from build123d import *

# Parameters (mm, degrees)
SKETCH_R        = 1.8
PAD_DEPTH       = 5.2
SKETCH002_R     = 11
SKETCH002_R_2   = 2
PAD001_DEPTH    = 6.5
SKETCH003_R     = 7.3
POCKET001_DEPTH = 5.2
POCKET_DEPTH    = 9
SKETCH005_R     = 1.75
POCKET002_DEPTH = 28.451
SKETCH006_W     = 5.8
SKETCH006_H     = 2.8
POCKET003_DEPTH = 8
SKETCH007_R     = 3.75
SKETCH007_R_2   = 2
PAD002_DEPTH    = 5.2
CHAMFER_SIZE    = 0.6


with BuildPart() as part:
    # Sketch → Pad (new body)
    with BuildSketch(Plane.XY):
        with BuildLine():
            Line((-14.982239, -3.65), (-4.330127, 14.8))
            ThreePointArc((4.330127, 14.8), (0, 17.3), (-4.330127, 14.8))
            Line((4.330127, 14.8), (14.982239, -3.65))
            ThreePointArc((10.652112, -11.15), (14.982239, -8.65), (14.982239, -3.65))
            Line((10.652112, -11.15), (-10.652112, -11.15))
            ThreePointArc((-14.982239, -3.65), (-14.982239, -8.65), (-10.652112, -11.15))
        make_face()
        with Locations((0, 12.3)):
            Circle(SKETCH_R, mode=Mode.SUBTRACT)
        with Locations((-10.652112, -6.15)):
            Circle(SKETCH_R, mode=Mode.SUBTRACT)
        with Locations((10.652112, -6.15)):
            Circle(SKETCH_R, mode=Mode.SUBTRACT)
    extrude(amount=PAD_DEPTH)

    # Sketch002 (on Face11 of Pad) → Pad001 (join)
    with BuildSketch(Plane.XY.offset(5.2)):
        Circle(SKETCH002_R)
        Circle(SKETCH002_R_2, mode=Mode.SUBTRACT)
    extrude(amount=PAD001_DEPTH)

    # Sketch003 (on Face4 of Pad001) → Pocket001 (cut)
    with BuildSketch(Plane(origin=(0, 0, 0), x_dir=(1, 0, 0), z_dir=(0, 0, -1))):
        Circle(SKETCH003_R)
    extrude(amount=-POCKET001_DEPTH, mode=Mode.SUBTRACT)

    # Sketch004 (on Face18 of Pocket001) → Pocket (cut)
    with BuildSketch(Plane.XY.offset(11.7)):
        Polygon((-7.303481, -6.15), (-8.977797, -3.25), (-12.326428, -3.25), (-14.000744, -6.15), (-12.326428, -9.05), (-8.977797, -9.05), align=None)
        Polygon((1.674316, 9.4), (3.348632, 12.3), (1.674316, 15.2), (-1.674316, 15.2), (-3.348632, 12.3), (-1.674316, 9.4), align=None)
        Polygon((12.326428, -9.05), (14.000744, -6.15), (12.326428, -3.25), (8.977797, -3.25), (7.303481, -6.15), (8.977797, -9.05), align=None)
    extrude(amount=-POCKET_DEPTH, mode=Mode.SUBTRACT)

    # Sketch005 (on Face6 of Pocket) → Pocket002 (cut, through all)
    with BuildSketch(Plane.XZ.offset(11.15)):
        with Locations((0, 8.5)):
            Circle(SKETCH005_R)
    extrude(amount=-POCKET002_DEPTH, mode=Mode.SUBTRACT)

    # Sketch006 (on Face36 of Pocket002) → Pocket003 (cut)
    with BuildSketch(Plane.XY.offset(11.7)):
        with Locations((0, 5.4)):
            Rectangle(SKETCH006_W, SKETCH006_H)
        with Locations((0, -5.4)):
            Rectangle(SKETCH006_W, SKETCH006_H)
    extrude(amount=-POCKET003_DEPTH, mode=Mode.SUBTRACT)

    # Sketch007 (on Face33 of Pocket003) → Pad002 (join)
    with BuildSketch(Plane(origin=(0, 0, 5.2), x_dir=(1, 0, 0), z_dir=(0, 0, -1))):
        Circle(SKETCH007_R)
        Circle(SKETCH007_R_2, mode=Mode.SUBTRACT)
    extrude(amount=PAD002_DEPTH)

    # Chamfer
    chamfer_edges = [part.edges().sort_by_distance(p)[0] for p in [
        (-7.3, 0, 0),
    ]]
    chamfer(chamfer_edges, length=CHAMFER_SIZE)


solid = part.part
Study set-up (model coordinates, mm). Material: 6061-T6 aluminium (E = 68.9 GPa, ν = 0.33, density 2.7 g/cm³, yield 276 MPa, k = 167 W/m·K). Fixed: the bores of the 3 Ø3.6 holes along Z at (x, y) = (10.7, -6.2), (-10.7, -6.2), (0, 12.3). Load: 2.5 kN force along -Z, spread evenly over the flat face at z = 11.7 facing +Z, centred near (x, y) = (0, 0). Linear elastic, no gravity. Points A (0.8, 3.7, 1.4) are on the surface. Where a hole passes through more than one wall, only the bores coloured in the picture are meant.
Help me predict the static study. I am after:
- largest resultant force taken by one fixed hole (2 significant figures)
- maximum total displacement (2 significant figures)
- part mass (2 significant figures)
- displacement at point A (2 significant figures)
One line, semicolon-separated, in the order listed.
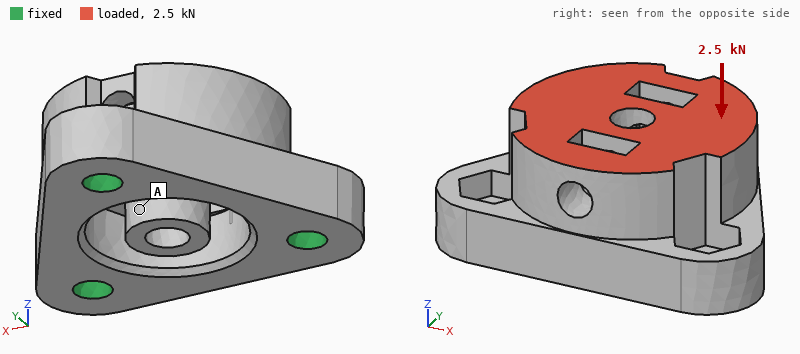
920 N; 8.2 µm; 11 g; 7.1 µm
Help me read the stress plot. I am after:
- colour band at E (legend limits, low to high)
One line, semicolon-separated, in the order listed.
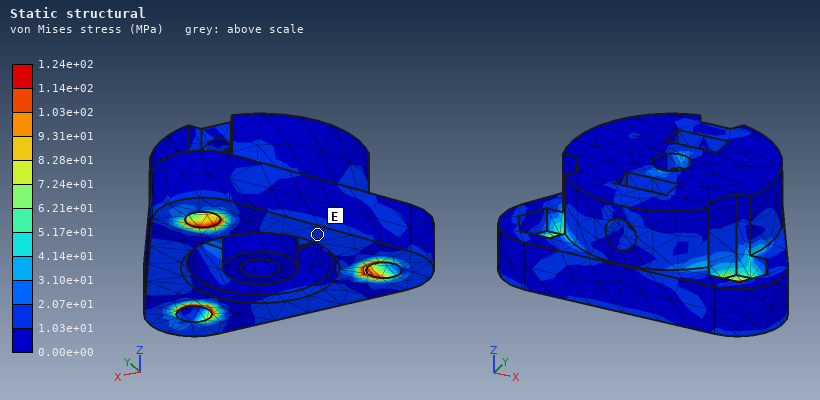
1.03e+01 to 2.07e+01 MPa
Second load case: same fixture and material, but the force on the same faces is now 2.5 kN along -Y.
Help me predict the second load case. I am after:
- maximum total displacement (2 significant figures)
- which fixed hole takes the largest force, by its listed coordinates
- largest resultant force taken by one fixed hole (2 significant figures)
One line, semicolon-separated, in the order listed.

23 µm; (0, 12.3); 1.7 kN
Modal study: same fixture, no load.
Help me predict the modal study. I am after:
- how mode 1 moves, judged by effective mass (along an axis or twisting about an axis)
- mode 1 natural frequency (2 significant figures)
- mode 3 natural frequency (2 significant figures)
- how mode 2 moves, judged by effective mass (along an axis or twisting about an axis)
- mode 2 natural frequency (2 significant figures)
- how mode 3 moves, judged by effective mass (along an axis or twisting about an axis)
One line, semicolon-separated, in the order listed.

along X; 29 kHz; 35 kHz; along Y; 31 kHz; along Z
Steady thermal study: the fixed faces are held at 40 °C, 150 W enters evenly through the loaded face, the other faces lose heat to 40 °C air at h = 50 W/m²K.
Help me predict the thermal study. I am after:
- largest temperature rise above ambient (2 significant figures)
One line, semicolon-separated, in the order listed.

67 K
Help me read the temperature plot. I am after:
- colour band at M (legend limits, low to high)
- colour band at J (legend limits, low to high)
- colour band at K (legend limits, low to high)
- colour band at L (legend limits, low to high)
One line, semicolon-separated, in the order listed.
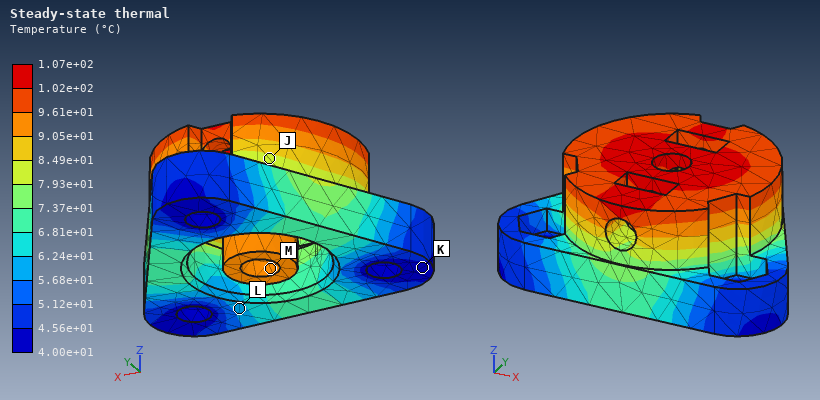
9.05e+01 to 9.61e+01 °C; 7.93e+01 to 8.49e+01 °C; 4.00e+01 to 4.56e+01 °C; 5.68e+01 to 6.24e+01 °C
